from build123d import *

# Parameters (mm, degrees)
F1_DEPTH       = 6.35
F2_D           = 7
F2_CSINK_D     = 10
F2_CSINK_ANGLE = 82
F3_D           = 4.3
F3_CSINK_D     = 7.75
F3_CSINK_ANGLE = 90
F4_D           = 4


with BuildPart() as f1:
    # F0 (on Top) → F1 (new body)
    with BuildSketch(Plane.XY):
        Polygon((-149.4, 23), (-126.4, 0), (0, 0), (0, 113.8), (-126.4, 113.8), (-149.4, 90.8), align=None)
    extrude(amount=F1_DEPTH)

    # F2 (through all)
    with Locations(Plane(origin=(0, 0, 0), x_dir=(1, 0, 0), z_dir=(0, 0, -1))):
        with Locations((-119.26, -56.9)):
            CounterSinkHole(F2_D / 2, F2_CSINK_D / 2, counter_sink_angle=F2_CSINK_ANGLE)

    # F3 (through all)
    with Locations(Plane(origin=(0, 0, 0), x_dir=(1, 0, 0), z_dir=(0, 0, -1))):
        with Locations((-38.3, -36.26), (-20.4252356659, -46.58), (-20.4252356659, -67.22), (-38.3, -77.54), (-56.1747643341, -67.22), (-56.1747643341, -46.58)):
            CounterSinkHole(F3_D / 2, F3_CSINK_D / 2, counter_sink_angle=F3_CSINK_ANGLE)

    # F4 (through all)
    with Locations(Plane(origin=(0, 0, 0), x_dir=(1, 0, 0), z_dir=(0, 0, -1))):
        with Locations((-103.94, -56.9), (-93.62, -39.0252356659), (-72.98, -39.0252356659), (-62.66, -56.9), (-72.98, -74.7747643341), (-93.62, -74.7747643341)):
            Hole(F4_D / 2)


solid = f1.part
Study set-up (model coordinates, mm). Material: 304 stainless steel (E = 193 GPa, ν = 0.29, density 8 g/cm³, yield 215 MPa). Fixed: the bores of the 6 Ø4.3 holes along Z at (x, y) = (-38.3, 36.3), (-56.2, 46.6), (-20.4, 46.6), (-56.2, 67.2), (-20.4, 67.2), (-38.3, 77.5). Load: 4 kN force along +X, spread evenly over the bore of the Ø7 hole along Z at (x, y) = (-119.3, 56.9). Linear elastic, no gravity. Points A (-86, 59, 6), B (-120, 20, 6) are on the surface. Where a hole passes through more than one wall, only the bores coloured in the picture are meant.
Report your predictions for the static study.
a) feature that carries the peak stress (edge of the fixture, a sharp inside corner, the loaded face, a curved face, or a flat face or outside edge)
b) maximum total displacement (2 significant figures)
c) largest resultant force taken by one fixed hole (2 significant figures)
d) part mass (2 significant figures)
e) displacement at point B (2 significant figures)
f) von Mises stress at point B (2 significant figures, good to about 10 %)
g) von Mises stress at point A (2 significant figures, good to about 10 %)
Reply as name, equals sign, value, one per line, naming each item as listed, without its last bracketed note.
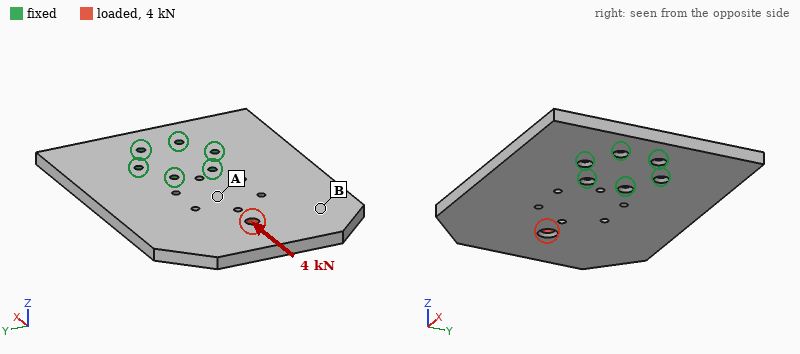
feature that carries the peak stress = the loaded face
maximum total displacement = 33 µm
largest resultant force taken by one fixed hole = 1.2 kN
part mass = 830 g
displacement at point B = 17 µm
von Mises stress at point B = 4.8 MPa
von Mises stress at point A = 16 MPa
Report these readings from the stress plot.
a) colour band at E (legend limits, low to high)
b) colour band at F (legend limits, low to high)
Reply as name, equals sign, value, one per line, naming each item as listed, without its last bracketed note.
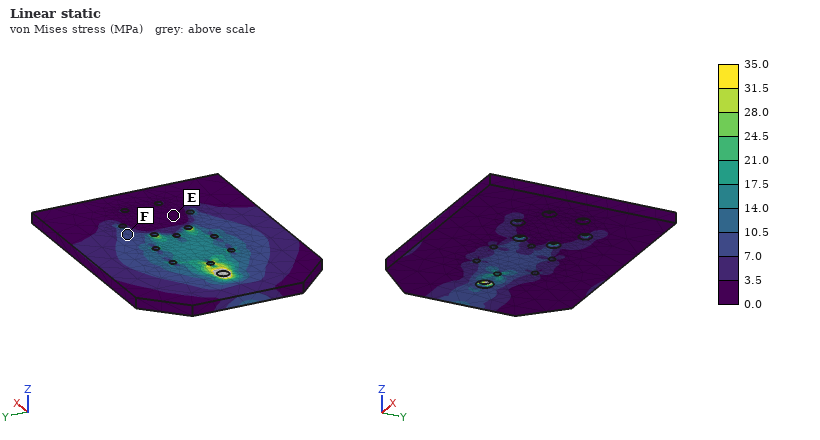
colour band at E = 0.0 to 3.5 MPa
colour band at F = 7.0 to 10.5 MPa
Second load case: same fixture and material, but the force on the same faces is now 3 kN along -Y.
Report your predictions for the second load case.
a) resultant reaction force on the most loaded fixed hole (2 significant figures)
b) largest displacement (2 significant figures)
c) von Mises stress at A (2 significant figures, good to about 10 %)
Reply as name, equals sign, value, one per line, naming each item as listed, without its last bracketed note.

resultant reaction force on the most loaded fixed hole = 2.6 kN
largest displacement = 20 µm
von Mises stress at A = 15 MPa
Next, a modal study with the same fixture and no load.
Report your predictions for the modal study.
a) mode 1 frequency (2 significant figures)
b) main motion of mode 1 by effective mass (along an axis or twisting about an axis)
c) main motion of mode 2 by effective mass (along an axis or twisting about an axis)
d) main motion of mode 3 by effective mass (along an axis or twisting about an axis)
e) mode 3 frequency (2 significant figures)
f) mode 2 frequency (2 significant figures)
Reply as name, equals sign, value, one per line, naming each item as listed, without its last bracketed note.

mode 1 frequency = 550 Hz
main motion of mode 1 by effective mass = along Z
main motion of mode 2 by effective mass = twisting about X
main motion of mode 3 by effective mass = along Z
mode 3 frequency = 2300 Hz
mode 2 frequency = 1000 Hz
